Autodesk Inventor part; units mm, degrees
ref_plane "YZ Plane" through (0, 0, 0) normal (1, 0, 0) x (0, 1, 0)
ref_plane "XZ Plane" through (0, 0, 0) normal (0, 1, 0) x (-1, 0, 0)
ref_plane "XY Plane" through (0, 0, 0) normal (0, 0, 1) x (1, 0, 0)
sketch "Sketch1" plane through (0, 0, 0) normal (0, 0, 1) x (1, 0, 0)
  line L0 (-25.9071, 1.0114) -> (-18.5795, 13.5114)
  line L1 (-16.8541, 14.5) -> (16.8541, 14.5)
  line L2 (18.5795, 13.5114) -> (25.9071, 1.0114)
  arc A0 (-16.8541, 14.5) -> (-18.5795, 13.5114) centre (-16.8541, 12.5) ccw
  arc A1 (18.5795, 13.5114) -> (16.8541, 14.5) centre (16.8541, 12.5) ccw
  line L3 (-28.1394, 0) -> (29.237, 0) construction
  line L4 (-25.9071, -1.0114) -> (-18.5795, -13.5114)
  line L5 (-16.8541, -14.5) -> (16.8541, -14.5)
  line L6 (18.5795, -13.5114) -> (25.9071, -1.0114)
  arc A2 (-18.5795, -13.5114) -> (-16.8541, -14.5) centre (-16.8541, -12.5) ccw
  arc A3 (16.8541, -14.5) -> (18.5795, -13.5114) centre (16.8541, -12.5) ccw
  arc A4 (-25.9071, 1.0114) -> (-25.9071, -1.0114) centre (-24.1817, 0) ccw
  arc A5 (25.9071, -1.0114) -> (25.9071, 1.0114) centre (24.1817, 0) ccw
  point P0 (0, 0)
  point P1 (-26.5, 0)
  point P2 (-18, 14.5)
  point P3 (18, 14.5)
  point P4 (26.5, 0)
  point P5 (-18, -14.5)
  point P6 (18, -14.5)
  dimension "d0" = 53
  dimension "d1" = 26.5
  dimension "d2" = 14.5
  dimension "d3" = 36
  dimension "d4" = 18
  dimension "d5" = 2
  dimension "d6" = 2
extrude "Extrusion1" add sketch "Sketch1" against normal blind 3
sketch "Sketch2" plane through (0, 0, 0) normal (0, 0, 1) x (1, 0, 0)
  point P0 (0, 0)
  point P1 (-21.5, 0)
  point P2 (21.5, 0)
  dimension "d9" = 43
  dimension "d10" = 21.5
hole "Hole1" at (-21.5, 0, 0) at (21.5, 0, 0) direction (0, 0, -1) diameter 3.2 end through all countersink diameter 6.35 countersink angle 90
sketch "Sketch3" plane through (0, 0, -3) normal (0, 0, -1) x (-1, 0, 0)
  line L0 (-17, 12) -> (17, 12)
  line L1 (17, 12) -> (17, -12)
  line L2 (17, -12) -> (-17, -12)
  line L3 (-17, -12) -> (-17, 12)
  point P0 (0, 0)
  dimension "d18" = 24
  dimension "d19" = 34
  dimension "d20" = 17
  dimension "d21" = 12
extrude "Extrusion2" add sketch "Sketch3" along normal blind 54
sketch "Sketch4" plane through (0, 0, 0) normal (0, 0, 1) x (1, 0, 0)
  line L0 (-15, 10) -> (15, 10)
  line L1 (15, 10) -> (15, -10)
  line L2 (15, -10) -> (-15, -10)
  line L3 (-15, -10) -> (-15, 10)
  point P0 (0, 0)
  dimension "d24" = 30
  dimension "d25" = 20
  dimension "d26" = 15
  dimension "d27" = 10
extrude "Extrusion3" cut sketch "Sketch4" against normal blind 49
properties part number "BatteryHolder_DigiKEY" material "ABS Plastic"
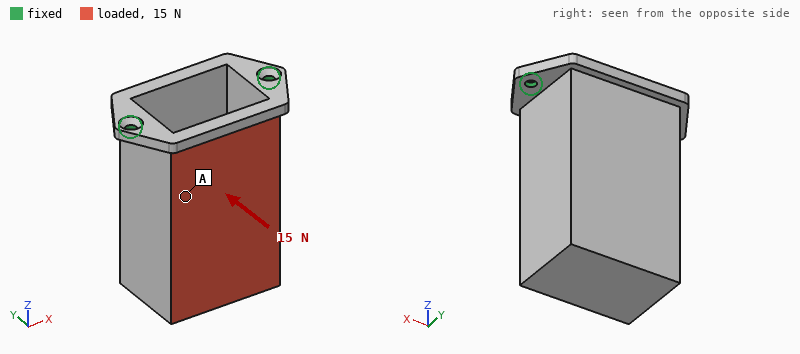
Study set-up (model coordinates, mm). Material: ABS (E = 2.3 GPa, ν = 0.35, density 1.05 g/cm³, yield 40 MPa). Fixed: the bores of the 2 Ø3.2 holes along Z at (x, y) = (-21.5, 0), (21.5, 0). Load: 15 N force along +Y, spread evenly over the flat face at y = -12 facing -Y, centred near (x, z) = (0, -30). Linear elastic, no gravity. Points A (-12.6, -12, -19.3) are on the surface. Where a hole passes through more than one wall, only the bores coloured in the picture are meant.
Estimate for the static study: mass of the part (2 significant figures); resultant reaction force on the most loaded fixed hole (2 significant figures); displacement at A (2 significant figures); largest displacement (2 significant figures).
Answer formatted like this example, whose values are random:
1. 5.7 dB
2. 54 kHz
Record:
1. 19 g
2. 7.6 N
3. 0.35 mm
4. 0.92 mm
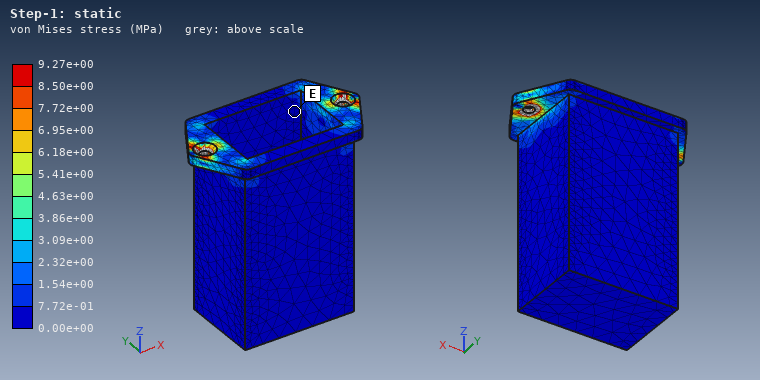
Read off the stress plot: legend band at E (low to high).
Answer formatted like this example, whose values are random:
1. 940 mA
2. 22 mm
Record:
1. 0.00e+00 to 7.72e-01 MPa
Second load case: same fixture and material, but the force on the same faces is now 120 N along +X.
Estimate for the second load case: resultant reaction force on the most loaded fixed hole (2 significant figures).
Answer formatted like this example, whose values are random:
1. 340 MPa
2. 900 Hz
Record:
1. 110 N
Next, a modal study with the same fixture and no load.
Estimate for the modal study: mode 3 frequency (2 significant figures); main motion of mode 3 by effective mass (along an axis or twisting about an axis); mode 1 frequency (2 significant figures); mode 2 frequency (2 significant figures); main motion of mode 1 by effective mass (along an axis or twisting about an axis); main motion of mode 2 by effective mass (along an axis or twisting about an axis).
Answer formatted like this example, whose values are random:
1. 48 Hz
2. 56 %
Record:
1. 1400 Hz
2. along Z
3. 160 Hz
4. 680 Hz
5. along Y
6. along X
